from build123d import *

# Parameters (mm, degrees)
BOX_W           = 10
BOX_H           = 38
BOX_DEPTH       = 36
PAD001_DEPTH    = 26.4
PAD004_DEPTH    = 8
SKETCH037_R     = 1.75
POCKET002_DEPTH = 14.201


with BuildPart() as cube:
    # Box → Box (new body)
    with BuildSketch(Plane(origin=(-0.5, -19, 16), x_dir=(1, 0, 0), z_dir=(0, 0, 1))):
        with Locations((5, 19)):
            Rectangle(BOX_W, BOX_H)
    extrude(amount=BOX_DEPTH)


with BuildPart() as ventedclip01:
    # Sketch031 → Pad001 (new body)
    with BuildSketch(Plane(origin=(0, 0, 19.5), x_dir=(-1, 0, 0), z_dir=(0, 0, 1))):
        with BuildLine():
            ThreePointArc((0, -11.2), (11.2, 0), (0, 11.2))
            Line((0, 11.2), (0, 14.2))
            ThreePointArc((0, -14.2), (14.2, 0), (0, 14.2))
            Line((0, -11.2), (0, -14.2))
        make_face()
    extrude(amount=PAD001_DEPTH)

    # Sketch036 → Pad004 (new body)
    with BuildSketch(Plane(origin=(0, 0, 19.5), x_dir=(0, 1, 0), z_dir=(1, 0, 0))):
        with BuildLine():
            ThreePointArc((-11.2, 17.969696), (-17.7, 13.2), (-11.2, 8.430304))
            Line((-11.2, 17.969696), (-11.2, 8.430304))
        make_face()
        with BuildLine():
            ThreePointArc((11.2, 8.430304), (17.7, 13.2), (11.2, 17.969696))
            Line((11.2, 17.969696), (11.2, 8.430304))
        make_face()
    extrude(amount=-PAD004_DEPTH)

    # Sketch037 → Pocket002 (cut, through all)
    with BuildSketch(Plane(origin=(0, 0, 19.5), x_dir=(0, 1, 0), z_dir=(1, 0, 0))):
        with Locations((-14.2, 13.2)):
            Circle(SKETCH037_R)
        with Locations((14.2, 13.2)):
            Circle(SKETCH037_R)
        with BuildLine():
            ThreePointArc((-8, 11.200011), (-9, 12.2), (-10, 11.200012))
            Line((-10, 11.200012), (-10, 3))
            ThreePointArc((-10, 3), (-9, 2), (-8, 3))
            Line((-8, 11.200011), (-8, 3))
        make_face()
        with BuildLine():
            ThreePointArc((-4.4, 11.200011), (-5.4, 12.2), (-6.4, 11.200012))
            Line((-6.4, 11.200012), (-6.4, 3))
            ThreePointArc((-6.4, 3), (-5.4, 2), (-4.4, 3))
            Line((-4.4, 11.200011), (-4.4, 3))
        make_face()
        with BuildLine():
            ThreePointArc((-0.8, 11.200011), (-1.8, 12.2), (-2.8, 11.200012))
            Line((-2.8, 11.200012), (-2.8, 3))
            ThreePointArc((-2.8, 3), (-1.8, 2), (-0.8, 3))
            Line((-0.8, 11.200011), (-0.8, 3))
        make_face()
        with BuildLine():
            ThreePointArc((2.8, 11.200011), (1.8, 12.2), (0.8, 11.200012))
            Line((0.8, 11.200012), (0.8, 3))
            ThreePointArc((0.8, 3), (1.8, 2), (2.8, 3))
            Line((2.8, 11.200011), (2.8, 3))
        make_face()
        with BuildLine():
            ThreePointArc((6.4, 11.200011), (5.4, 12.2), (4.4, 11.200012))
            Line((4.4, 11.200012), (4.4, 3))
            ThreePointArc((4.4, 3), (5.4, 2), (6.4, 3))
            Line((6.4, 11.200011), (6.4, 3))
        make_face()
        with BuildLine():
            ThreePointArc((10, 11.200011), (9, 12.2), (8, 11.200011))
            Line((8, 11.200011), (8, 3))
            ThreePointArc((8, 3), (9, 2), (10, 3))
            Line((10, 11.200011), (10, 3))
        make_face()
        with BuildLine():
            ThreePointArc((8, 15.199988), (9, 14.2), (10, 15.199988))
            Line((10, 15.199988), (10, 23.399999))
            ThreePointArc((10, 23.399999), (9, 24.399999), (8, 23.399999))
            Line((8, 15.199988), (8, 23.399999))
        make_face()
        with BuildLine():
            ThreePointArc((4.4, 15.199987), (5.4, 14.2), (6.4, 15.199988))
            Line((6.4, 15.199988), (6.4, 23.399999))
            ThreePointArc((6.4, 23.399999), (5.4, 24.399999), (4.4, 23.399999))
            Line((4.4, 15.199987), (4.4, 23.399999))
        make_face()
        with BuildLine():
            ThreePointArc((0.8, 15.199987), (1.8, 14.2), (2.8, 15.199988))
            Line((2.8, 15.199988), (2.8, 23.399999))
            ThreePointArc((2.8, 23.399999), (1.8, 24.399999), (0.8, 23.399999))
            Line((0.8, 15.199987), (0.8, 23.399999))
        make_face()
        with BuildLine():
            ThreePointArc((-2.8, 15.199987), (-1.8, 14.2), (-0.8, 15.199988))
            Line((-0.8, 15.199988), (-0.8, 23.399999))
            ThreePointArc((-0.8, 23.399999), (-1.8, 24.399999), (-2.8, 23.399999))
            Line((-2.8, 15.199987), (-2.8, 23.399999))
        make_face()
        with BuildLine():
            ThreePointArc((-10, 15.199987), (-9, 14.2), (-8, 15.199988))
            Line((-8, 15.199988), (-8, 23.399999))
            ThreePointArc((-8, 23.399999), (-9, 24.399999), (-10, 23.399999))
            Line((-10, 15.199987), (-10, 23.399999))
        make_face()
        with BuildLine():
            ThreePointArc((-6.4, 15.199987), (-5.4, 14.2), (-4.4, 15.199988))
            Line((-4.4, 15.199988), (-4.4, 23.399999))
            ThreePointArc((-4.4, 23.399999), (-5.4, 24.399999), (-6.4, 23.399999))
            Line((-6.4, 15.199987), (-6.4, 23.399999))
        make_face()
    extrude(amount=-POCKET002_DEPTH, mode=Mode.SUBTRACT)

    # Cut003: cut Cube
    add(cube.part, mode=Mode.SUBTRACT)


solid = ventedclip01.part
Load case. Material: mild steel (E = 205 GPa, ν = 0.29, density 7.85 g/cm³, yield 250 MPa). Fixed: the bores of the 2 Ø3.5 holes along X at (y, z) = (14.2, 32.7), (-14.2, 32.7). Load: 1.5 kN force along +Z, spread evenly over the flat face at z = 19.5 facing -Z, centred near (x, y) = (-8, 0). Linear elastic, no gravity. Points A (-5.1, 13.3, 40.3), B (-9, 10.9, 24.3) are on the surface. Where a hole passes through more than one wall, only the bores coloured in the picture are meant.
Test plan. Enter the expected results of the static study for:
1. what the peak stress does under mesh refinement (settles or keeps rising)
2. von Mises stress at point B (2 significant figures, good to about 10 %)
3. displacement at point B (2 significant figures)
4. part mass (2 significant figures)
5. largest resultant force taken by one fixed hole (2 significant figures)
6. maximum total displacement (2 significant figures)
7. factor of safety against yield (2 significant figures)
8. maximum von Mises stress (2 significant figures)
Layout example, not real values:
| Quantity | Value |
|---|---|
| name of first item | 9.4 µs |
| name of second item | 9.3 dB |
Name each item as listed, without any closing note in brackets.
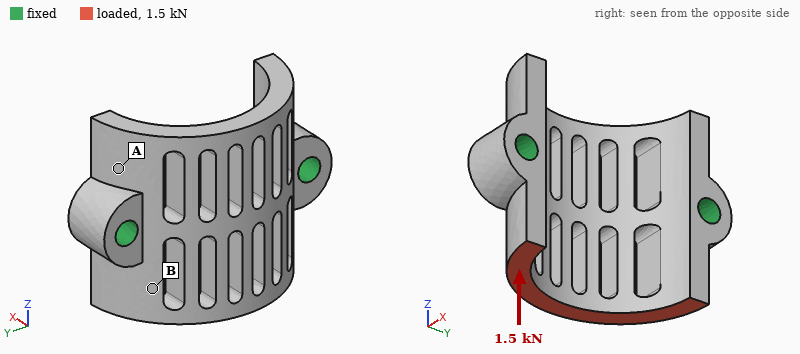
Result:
| Quantity | Value |
|---|---|
| what the peak stress does under mesh refinement | settles |
| von Mises stress at point B | 53 MPa |
| displacement at point B | 3.2 µm |
| part mass | 20 g |
| largest resultant force taken by one fixed hole | 750 N |
| maximum total displacement | 16 µm |
| factor of safety against yield | 1.4 |
| maximum von Mises stress | 180 MPa |
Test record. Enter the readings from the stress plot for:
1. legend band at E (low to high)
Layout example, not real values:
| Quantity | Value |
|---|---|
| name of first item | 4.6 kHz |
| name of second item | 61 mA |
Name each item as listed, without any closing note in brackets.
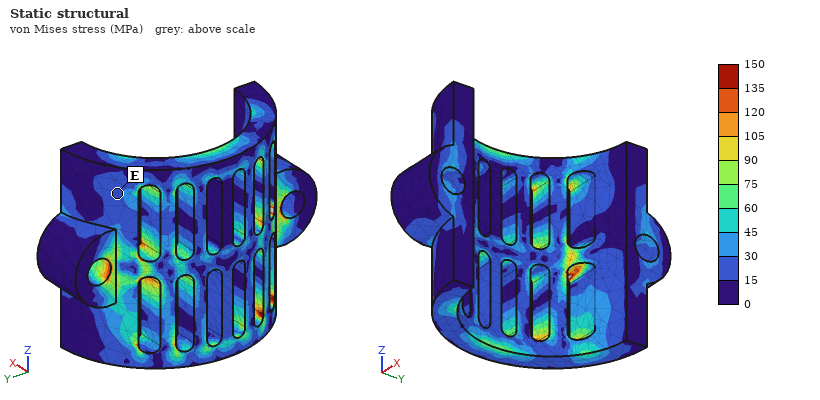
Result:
| Quantity | Value |
|---|---|
| legend band at E | 15 to 30 MPa |
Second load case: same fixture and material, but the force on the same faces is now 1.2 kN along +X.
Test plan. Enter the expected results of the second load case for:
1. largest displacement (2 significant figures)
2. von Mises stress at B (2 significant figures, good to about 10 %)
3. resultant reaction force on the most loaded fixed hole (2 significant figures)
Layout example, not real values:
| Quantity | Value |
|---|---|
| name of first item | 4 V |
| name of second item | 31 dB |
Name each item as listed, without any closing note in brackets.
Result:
| Quantity | Value |
|---|---|
| largest displacement | 27 µm |
| von Mises stress at B | 79 MPa |
| resultant reaction force on the most loaded fixed hole | 660 N |
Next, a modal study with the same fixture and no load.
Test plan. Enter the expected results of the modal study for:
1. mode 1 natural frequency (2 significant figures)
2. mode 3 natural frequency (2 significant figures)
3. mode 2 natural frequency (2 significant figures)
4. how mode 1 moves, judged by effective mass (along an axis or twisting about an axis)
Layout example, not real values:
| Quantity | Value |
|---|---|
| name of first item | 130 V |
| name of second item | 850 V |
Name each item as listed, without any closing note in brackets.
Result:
| Quantity | Value |
|---|---|
| mode 1 natural frequency | 15 kHz |
| mode 3 natural frequency | 17 kHz |
| mode 2 natural frequency | 17 kHz |
| how mode 1 moves, judged by effective mass | along Z |
